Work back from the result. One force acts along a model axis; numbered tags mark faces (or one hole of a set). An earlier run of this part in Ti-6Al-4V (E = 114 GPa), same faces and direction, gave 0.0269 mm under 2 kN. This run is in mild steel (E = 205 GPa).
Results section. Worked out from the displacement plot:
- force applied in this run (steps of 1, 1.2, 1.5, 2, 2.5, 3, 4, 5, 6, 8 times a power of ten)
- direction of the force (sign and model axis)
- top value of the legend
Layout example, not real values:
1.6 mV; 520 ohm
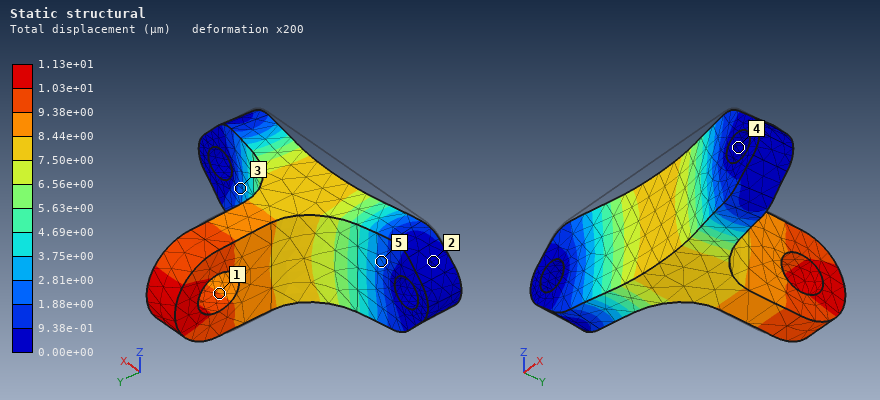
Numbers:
1.5 kN; +Y; 1.13e+01 µm
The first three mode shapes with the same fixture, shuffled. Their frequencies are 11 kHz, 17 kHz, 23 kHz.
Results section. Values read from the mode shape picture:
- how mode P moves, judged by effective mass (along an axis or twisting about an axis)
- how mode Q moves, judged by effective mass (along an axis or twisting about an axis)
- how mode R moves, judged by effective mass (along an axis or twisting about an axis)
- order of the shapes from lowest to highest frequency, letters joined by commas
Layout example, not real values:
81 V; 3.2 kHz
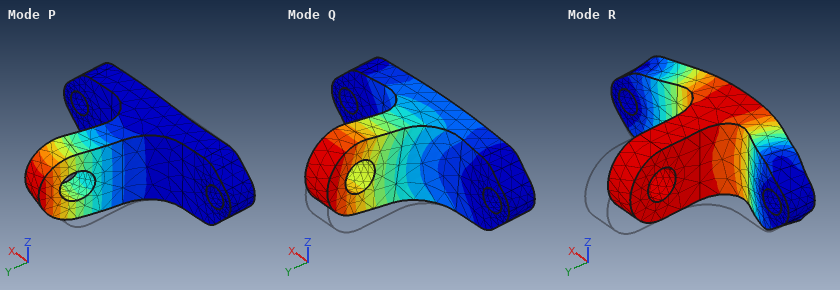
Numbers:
along X; along Z; along Y; Q, P, R
